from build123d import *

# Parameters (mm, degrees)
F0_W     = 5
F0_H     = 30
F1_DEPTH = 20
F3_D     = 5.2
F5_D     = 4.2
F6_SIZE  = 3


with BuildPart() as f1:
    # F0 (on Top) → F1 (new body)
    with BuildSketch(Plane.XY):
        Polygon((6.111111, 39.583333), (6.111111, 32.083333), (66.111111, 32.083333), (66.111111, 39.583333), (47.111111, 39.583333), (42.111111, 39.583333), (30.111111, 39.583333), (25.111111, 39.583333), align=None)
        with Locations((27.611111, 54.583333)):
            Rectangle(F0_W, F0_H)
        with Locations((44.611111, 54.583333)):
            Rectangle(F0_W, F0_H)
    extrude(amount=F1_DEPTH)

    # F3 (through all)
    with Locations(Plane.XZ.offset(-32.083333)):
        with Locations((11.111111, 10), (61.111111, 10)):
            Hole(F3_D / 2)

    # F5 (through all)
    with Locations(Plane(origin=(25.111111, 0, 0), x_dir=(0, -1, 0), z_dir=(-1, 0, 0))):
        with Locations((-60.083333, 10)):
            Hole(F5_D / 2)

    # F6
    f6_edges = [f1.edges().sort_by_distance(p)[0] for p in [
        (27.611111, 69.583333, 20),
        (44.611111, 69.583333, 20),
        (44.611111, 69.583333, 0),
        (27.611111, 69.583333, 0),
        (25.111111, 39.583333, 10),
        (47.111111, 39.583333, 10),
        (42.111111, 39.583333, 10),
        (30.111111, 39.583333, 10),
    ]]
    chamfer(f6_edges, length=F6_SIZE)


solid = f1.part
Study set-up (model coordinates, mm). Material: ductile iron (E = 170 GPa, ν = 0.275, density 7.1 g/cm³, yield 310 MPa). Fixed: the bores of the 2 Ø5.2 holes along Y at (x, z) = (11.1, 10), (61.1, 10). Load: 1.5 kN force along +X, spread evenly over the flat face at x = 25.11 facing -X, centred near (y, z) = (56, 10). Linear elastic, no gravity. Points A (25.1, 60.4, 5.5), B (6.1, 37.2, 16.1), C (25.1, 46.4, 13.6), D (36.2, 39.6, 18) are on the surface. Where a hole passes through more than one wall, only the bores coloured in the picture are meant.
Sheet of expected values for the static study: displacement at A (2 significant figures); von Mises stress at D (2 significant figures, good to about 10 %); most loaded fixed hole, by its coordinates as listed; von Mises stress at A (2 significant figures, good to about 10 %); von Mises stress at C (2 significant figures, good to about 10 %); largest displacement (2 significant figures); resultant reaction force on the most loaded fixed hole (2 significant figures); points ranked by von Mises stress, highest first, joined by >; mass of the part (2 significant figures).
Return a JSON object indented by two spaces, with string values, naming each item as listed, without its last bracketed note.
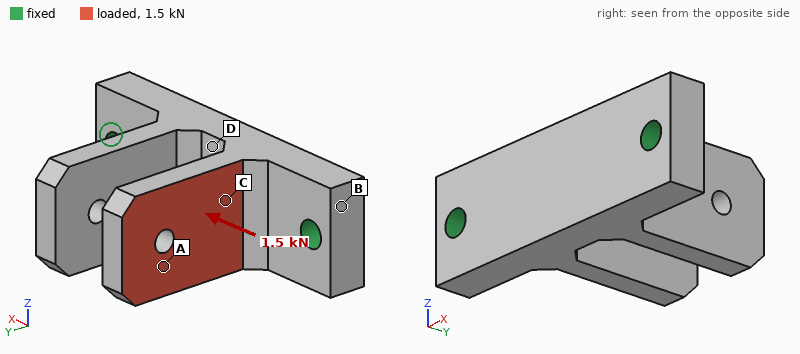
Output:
{
  "displacement at A": "0.096 mm",
  "von Mises stress at D": "56 MPa",
  "most loaded fixed hole, by its coordinates as listed": "(11.1, 10)",
  "von Mises stress at A": "33 MPa",
  "von Mises stress at C": "160 MPa",
  "largest displacement": "0.16 mm",
  "resultant reaction force on the most loaded fixed hole": "1.2 kN",
  "points ranked by von Mises stress, highest first, joined by >": "C > D > A > B",
  "mass of the part": "110 g"
}
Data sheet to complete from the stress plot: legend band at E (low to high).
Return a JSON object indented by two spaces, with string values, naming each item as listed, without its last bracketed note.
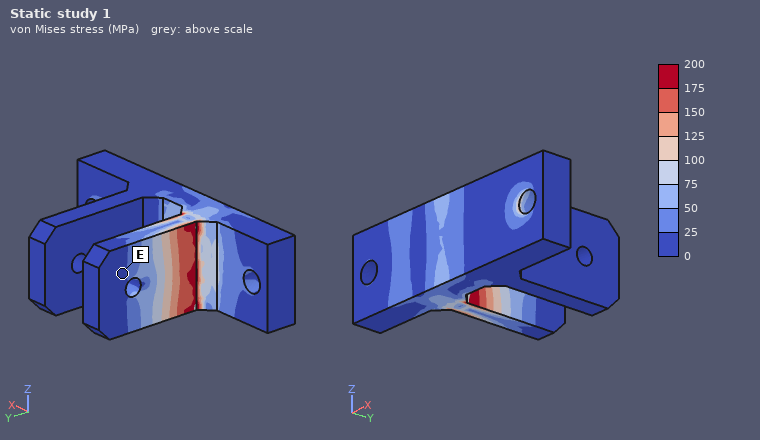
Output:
{
  "legend band at E": "0 to 25 MPa"
}
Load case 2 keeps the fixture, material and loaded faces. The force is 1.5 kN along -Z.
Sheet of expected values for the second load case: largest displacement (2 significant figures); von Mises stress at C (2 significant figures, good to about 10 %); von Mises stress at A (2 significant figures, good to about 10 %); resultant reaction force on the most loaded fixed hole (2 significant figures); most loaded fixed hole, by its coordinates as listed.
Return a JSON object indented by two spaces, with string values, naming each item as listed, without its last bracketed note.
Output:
{
  "largest displacement": "75 µm",
  "von Mises stress at C": "57 MPa",
  "von Mises stress at A": "36 MPa",
  "resultant reaction force on the most loaded fixed hole": "1.1 kN",
  "most loaded fixed hole, by its coordinates as listed": "(11.1, 10)"
}
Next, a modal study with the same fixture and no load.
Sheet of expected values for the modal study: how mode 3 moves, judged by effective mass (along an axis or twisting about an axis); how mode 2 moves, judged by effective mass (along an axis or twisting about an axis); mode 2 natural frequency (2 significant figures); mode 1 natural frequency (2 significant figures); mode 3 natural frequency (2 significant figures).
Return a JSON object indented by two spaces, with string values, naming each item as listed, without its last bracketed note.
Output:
{
  "how mode 3 moves, judged by effective mass": "along Z",
  "how mode 2 moves, judged by effective mass": "along X",
  "mode 2 natural frequency": "4700 Hz",
  "mode 1 natural frequency": "4300 Hz",
  "mode 3 natural frequency": "5000 Hz"
}
